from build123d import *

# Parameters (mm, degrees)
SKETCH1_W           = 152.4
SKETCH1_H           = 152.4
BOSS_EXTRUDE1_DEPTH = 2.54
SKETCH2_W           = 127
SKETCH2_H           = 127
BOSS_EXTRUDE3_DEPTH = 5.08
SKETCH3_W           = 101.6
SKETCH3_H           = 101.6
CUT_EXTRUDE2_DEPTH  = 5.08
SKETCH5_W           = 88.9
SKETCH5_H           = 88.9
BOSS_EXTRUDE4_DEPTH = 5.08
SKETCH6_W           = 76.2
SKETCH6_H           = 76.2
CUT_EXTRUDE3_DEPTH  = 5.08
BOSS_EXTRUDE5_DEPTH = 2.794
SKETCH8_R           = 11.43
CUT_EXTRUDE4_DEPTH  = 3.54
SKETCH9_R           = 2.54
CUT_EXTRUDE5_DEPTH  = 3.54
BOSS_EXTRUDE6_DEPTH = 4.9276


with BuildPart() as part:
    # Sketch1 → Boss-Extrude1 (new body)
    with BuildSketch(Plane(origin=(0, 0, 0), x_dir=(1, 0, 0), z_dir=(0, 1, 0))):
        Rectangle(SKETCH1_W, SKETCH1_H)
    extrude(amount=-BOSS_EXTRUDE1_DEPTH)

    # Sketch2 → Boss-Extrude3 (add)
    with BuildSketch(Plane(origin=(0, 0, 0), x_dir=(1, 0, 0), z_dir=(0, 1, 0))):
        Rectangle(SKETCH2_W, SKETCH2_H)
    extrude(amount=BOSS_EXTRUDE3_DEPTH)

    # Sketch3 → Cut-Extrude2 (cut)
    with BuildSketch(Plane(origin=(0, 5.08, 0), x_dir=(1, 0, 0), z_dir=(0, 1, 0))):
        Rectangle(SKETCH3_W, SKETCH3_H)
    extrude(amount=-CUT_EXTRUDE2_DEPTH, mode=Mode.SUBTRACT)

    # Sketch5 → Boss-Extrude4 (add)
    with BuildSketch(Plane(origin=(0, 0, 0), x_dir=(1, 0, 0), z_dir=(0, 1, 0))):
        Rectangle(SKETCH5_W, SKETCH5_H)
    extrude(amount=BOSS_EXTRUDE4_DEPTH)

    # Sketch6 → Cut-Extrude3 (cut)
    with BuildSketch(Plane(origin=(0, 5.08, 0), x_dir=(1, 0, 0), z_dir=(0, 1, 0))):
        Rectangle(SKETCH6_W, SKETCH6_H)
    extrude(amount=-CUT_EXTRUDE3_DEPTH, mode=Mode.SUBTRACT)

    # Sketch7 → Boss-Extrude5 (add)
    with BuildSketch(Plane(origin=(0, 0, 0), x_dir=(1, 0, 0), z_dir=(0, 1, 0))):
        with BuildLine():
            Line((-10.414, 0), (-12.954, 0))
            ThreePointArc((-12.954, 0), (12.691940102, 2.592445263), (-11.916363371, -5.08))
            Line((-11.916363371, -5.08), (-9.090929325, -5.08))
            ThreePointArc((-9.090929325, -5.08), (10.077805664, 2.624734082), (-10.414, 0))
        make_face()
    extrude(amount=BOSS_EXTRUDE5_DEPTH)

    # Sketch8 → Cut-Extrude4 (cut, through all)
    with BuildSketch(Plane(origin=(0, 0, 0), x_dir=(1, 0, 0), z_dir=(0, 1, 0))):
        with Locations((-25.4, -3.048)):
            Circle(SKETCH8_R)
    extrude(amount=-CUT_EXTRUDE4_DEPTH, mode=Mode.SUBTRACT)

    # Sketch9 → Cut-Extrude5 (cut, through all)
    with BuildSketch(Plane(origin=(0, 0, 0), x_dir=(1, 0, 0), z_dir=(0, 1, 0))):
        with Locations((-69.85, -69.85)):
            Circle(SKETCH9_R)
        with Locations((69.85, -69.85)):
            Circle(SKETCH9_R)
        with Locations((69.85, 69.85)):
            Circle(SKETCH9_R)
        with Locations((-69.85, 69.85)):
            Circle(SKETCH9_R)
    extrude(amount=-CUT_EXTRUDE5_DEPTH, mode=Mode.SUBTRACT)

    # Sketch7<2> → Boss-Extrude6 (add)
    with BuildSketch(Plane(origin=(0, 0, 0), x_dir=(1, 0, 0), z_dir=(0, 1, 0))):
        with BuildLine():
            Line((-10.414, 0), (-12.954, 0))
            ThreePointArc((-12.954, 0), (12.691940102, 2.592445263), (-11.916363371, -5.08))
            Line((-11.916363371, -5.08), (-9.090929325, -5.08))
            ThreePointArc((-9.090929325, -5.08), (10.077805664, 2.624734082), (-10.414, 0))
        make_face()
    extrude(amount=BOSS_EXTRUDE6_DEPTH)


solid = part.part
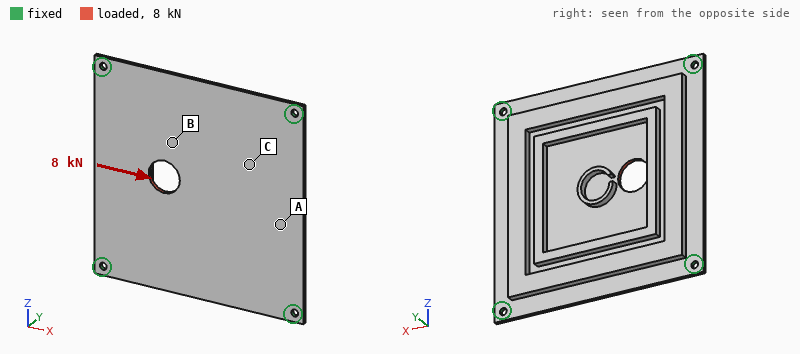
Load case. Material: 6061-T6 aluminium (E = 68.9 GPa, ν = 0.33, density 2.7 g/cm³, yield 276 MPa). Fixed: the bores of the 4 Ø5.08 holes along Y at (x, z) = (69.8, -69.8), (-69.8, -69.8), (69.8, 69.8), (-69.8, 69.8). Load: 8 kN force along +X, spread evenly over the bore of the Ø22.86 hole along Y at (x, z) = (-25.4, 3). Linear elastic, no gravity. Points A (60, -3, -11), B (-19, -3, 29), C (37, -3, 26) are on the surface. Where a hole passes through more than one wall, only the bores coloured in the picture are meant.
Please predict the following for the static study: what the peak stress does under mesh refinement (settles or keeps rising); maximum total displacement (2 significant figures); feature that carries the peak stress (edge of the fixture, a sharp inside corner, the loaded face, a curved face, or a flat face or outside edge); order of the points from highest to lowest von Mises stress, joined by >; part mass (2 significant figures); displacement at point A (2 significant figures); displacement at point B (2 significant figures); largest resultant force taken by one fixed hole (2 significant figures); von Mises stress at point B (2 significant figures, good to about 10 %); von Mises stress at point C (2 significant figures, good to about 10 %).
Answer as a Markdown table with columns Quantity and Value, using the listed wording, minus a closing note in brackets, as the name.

| Quantity | Value |
|---|---|
| what the peak stress does under mesh refinement | keeps rising |
| maximum total displacement | 75 µm |
| feature that carries the peak stress | edge of the fixture |
| order of the points from highest to lowest von Mises stress, joined by > | B > C > A |
| part mass | 270 g |
| displacement at point A | 39 µm |
| displacement at point B | 35 µm |
| largest resultant force taken by one fixed hole | 2.4 kN |
| von Mises stress at point B | 28 MPa |
| von Mises stress at point C | 16 MPa |
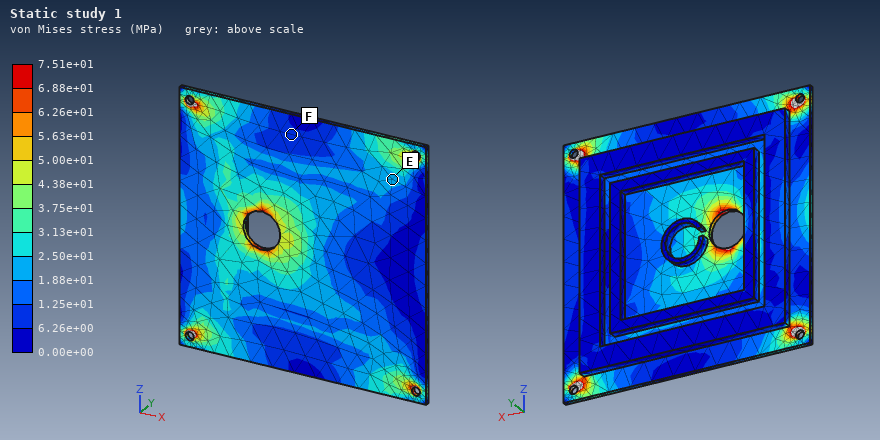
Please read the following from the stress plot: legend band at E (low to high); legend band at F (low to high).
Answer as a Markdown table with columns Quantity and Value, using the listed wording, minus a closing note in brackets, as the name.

| Quantity | Value |
|---|---|
| legend band at E | 1.88e+01 to 2.50e+01 MPa |
| legend band at F | 6.26e+00 to 1.25e+01 MPa |
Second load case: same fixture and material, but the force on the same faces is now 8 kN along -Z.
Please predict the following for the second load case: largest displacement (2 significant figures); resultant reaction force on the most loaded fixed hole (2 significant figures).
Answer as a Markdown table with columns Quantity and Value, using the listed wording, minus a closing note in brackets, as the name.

| Quantity | Value |
|---|---|
| largest displacement | 52 µm |
| resultant reaction force on the most loaded fixed hole | 2.7 kN |
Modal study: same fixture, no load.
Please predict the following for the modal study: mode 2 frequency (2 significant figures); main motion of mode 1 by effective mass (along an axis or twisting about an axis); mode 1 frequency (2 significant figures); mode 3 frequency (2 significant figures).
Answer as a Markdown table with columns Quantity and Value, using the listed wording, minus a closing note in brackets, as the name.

| Quantity | Value |
|---|---|
| mode 2 frequency | 1300 Hz |
| main motion of mode 1 by effective mass | along Y |
| mode 1 frequency | 760 Hz |
| mode 3 frequency | 1300 Hz |
